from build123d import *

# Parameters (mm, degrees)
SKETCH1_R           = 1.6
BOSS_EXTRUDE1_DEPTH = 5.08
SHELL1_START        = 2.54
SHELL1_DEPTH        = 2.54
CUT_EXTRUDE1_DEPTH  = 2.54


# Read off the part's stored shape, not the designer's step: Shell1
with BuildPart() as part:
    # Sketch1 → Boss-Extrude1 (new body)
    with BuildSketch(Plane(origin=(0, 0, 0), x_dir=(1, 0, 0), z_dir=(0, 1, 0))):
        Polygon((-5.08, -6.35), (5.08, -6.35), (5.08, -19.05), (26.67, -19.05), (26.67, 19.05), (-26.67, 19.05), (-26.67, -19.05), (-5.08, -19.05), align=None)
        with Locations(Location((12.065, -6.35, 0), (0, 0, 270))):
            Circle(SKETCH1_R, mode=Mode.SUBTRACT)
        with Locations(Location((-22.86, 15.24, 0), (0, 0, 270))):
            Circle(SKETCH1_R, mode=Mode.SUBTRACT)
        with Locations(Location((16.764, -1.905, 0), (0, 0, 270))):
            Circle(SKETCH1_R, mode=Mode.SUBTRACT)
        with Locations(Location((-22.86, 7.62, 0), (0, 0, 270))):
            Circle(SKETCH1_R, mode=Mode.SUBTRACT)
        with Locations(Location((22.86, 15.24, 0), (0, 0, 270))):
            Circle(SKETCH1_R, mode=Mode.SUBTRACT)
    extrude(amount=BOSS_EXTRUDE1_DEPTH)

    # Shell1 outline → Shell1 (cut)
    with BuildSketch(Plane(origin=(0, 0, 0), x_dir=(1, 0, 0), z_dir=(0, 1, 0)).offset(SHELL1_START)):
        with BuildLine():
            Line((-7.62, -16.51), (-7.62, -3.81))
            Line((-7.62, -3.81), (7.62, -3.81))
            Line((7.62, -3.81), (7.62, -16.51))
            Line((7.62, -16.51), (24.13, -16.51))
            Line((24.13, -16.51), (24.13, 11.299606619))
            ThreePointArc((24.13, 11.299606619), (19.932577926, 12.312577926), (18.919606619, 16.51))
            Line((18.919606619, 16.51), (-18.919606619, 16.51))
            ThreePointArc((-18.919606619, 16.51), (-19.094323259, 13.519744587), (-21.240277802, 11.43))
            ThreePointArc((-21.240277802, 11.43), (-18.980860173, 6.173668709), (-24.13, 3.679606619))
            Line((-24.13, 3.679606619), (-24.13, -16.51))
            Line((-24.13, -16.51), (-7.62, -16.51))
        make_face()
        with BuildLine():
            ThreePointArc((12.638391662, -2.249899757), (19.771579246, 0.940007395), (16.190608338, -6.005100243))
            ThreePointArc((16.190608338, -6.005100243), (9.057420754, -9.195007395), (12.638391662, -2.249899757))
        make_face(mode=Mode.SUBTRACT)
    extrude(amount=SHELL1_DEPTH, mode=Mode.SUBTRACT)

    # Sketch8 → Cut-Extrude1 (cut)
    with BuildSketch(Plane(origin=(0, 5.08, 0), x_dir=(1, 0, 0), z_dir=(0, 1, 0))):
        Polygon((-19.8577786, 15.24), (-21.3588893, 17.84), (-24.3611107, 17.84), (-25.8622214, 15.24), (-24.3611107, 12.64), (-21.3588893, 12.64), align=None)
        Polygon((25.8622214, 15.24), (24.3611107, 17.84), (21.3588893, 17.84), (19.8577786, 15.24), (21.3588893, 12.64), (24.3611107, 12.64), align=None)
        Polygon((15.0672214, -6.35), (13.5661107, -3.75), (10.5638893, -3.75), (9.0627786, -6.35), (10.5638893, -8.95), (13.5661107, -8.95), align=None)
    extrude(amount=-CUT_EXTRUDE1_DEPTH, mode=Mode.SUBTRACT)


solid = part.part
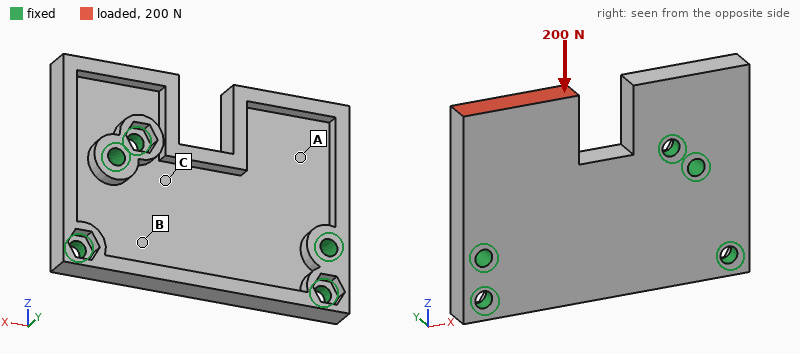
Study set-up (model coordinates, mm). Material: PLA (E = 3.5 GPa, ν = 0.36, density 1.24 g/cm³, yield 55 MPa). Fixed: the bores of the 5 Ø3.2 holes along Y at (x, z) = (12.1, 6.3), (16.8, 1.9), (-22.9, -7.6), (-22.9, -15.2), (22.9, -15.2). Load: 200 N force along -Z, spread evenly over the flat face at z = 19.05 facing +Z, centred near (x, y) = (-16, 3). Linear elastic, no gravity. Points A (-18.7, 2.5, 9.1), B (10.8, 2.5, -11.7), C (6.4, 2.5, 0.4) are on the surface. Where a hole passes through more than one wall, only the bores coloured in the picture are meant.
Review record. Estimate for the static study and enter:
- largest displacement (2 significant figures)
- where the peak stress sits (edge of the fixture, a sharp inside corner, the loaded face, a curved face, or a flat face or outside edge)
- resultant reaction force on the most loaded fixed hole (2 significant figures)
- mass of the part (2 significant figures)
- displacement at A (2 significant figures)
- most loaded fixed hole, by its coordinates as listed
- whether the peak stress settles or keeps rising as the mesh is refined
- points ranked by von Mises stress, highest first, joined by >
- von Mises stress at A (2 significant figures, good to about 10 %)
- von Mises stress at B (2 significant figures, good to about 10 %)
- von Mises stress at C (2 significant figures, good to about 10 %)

0.23 mm
a sharp inside corner
130 N
7.8 g
0.076 mm
(-22.9, -7.6)
keeps rising
A > C > B
5.7 MPa
1.0 MPa
2.9 MPa
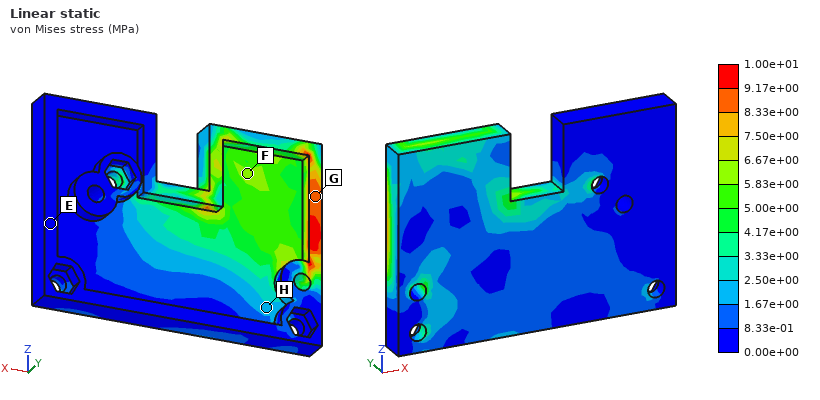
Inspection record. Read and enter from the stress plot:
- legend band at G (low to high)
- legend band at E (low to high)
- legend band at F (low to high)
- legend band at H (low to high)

8.33e+00 to 9.17e+00 MPa
0.00e+00 to 8.33e-01 MPa
5.83e+00 to 6.67e+00 MPa
1.67e+00 to 2.50e+00 MPa
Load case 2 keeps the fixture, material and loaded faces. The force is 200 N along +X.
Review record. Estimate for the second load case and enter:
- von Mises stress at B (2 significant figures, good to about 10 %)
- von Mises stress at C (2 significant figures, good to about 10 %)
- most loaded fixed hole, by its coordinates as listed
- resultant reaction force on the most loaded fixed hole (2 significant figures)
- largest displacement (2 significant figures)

3.4 MPa
6.6 MPa
(-22.9, -7.6)
160 N
0.33 mm
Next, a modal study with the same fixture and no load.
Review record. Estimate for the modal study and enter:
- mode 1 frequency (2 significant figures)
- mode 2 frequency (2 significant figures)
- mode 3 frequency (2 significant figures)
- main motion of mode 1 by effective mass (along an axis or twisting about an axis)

1400 Hz
3200 Hz
3500 Hz
along Y
